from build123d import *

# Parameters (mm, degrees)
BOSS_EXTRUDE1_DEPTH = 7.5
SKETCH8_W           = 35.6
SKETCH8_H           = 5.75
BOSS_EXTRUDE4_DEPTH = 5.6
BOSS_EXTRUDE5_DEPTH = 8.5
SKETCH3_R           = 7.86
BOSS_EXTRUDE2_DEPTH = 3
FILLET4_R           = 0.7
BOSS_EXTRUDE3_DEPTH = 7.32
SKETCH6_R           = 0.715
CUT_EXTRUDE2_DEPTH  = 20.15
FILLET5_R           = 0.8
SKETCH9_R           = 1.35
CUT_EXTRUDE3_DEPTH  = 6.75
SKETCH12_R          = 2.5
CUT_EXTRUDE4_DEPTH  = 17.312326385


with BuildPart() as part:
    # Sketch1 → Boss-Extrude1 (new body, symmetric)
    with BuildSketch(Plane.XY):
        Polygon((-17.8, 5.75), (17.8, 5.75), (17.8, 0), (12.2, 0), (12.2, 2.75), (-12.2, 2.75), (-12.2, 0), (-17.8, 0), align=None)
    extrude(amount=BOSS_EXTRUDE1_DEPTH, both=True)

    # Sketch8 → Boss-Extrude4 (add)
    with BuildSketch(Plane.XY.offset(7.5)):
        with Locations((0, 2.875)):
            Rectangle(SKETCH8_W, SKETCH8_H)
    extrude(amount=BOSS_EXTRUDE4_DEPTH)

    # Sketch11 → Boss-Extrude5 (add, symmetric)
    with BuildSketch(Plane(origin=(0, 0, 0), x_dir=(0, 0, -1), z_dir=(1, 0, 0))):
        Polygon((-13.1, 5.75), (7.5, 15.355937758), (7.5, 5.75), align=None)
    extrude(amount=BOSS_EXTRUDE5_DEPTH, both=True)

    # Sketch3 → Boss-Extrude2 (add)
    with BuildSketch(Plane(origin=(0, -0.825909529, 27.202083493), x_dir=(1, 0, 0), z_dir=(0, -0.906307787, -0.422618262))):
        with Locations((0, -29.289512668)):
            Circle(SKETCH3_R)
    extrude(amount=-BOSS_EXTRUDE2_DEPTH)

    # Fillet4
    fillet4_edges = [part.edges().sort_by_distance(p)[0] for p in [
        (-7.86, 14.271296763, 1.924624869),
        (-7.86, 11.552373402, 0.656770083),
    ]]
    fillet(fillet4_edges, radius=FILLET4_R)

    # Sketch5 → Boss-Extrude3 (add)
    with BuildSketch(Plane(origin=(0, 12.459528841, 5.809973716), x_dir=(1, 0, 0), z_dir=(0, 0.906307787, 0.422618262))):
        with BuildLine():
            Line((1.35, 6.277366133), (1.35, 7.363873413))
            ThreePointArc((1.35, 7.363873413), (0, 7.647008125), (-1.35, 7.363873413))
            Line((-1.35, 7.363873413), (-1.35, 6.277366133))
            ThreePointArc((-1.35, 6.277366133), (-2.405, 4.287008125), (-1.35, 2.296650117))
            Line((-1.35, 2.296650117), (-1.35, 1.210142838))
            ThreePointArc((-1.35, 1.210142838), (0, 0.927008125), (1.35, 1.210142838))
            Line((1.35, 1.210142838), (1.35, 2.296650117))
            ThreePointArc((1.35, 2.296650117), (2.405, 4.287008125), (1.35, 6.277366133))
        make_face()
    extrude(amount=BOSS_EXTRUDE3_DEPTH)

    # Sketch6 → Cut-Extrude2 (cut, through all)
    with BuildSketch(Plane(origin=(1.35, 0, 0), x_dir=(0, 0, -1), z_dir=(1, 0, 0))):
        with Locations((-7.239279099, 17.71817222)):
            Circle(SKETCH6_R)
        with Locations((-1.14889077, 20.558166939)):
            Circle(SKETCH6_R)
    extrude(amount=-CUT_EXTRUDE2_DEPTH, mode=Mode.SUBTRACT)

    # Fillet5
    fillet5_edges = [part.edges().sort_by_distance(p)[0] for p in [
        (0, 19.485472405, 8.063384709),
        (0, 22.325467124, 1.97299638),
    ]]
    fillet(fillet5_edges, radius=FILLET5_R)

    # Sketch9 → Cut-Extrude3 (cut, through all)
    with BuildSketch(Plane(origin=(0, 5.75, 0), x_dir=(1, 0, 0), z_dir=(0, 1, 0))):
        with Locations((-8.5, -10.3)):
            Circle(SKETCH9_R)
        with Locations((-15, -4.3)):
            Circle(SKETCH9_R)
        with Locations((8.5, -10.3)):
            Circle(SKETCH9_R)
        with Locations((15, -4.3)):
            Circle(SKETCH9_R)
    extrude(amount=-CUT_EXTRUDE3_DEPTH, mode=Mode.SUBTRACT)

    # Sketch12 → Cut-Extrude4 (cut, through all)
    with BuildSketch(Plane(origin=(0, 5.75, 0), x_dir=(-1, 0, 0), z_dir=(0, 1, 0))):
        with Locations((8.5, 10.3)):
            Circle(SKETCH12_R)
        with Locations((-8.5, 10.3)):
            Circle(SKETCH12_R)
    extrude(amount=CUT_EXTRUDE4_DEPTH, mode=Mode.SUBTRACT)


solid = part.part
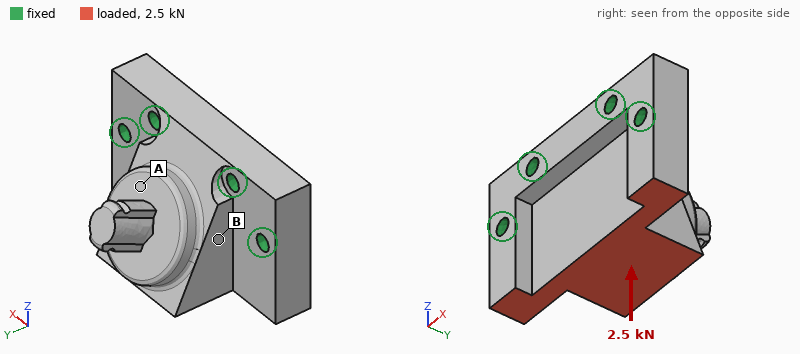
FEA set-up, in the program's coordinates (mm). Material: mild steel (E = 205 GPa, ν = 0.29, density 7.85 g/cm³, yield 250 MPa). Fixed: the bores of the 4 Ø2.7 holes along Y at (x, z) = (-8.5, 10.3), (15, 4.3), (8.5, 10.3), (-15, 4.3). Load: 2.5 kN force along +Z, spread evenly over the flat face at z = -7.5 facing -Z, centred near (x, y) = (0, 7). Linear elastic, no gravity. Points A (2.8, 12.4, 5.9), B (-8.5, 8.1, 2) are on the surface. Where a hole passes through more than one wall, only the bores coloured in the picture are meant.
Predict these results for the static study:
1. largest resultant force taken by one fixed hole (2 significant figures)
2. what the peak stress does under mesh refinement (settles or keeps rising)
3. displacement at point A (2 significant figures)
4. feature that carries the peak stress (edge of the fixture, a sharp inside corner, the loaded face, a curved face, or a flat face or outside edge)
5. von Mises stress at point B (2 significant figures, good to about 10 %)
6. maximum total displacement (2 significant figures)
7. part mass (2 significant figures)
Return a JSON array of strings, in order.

["960 N", "keeps rising", "5.4 µm", "edge of the fixture", "21 MPa", "11 µm", "43 g"]
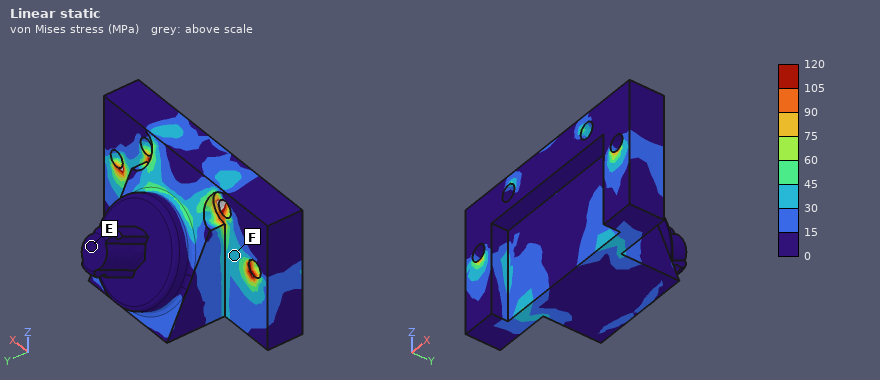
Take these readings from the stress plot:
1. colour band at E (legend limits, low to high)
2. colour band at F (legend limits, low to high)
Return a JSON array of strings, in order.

["0 to 15 MPa", "30 to 45 MPa"]
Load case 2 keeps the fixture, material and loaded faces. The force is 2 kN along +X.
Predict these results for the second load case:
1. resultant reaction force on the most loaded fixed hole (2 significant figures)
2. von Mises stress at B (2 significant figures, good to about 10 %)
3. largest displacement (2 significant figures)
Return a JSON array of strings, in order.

["940 N", "15 MPa", "4.2 µm"]
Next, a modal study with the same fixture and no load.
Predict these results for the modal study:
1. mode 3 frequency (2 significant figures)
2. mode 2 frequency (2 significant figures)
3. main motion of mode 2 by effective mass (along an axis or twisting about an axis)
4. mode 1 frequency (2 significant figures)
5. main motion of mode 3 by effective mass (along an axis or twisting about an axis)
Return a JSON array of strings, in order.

["37 kHz", "26 kHz", "along X", "12 kHz", "along X"]
